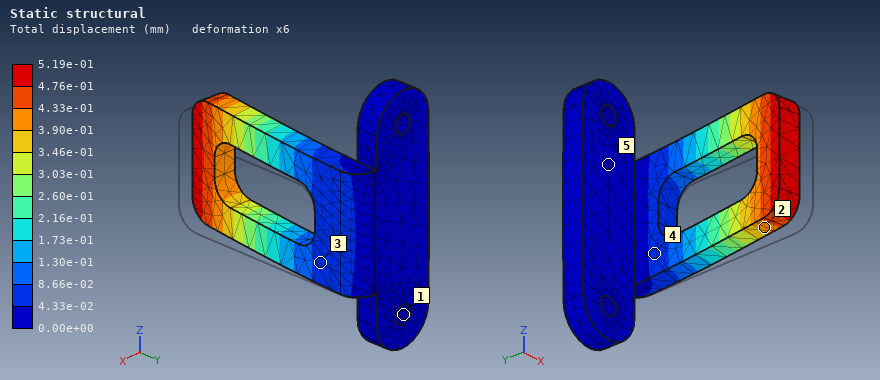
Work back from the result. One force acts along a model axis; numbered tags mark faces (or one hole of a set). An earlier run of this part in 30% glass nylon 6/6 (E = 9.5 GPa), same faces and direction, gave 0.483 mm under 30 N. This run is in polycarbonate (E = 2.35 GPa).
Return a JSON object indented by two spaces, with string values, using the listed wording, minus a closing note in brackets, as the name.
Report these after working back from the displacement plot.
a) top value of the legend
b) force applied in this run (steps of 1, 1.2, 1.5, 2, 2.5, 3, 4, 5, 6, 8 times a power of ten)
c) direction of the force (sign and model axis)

{
  "top value of the legend": "5.19e-01 mm",
  "force applied in this run": "8 N",
  "direction of the force": "-X"
}
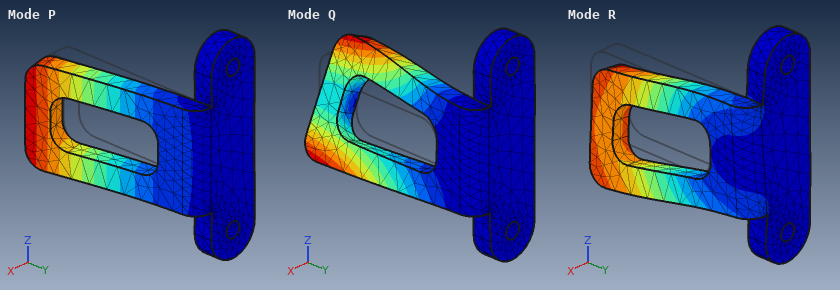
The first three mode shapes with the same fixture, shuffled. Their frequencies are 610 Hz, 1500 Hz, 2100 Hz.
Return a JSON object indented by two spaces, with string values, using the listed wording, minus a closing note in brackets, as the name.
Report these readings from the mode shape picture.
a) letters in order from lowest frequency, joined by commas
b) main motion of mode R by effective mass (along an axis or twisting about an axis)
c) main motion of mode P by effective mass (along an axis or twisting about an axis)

{
  "letters in order from lowest frequency, joined by commas": "P, R, Q",
  "main motion of mode R by effective mass": "along Z",
  "main motion of mode P by effective mass": "along X"
}
